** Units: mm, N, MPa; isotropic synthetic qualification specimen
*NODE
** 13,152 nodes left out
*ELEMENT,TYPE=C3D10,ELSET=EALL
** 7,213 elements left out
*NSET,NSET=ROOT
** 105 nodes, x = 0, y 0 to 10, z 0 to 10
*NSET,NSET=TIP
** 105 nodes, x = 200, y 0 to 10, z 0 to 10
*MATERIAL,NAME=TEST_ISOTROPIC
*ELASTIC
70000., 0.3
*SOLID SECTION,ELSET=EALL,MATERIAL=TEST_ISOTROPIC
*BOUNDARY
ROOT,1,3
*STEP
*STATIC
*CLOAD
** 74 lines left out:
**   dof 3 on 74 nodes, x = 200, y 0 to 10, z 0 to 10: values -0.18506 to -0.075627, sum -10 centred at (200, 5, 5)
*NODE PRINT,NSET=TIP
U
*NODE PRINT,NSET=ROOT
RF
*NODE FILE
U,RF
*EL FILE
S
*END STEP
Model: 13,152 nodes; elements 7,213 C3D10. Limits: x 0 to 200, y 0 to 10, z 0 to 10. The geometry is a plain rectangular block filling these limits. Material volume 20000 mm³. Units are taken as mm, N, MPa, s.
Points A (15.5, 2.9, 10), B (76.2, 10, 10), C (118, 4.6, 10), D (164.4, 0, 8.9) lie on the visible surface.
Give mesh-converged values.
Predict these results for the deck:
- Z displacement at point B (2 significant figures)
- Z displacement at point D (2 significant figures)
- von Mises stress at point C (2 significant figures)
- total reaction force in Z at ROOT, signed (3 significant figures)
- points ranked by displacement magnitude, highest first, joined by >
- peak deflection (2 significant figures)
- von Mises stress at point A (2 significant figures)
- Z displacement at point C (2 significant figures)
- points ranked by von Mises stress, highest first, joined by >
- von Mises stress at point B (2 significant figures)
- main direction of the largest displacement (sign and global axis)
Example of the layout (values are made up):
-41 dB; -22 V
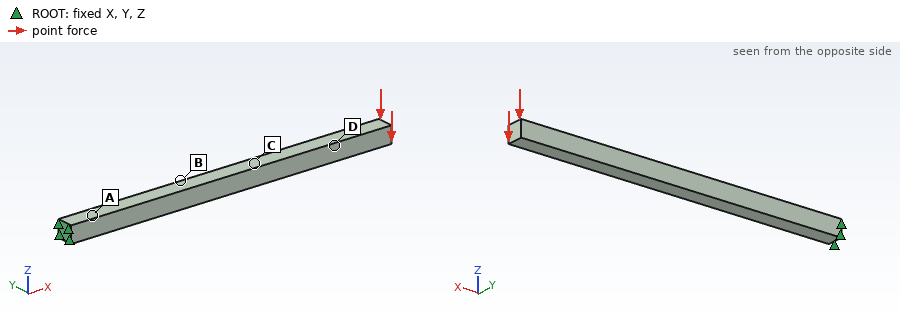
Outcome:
-0.087 mm; -0.34 mm; 4.9 MPa; 10.0 N; D > C > B > A; 0.46 mm; 11 MPa; -0.19 mm; A > B > C > D; 7.4 MPa; -Z
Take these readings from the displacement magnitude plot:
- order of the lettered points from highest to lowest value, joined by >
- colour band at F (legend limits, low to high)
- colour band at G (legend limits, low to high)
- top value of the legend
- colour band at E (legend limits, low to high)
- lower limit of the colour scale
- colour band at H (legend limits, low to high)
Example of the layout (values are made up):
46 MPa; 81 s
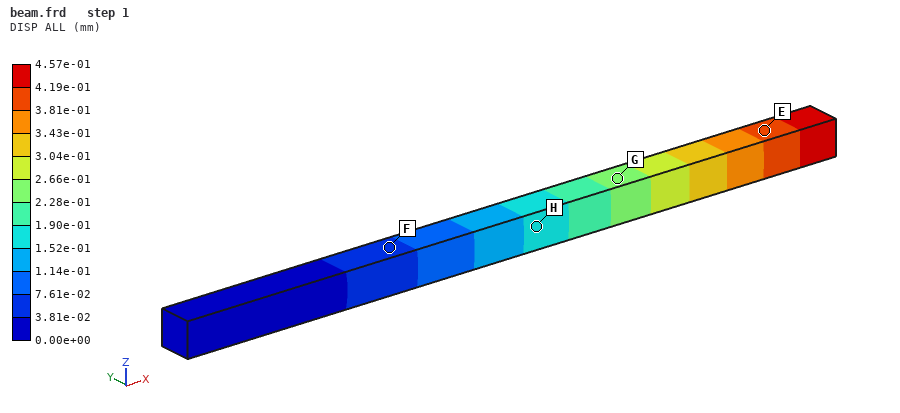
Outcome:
E > G > H > F; 3.81e-02 to 7.61e-02 mm; 2.28e-01 to 2.66e-01 mm; 4.57e-01 mm; 3.81e-01 to 4.19e-01 mm; 0.00e+00 mm; 1.52e-01 to 1.90e-01 mm
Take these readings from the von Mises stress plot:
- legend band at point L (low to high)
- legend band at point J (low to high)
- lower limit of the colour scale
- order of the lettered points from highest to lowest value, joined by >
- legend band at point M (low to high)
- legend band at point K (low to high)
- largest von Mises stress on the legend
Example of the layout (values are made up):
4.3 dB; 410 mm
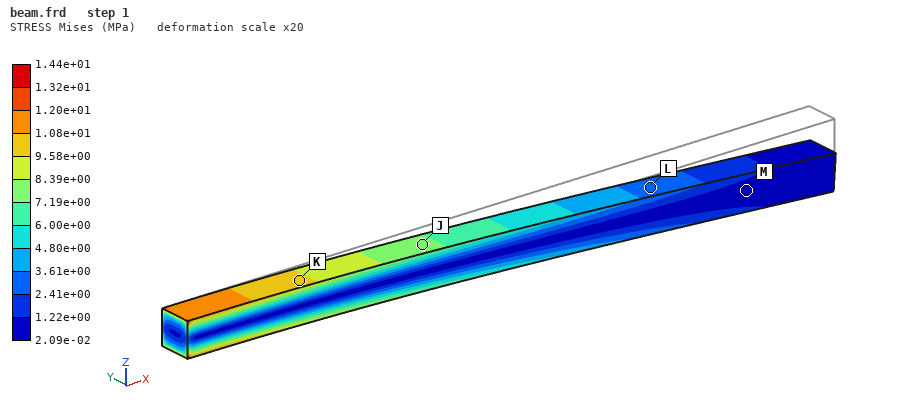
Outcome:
2.41e+00 to 3.61e+00 MPa; 7.19e+00 to 8.39e+00 MPa; 2.09e-02 MPa; K > J > L > M; 2.09e-02 to 1.22e+00 MPa; 9.58e+00 to 1.08e+01 MPa; 1.44e+01 MPa
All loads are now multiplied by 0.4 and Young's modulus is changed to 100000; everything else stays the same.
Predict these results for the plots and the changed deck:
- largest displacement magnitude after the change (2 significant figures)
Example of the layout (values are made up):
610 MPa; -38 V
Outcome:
0.13 mm
